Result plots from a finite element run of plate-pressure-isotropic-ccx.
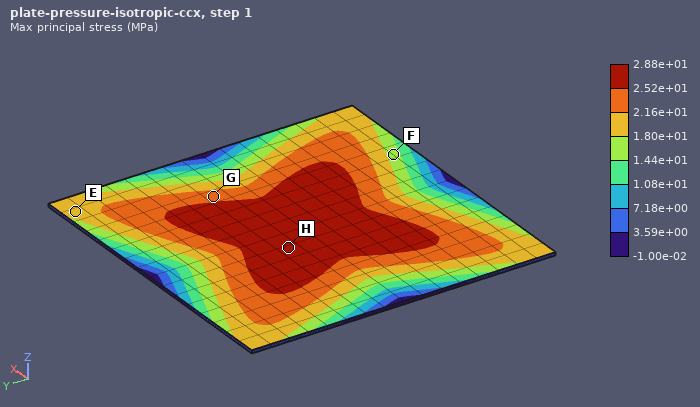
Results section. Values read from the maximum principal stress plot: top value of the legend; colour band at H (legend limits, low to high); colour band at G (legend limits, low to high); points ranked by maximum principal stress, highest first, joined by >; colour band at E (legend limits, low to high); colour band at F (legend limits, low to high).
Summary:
2.88e+01 MPa
2.52e+01 to 2.88e+01 MPa
2.16e+01 to 2.52e+01 MPa
H > G > E > F
1.80e+01 to 2.16e+01 MPa
1.44e+01 to 1.80e+01 MPa
